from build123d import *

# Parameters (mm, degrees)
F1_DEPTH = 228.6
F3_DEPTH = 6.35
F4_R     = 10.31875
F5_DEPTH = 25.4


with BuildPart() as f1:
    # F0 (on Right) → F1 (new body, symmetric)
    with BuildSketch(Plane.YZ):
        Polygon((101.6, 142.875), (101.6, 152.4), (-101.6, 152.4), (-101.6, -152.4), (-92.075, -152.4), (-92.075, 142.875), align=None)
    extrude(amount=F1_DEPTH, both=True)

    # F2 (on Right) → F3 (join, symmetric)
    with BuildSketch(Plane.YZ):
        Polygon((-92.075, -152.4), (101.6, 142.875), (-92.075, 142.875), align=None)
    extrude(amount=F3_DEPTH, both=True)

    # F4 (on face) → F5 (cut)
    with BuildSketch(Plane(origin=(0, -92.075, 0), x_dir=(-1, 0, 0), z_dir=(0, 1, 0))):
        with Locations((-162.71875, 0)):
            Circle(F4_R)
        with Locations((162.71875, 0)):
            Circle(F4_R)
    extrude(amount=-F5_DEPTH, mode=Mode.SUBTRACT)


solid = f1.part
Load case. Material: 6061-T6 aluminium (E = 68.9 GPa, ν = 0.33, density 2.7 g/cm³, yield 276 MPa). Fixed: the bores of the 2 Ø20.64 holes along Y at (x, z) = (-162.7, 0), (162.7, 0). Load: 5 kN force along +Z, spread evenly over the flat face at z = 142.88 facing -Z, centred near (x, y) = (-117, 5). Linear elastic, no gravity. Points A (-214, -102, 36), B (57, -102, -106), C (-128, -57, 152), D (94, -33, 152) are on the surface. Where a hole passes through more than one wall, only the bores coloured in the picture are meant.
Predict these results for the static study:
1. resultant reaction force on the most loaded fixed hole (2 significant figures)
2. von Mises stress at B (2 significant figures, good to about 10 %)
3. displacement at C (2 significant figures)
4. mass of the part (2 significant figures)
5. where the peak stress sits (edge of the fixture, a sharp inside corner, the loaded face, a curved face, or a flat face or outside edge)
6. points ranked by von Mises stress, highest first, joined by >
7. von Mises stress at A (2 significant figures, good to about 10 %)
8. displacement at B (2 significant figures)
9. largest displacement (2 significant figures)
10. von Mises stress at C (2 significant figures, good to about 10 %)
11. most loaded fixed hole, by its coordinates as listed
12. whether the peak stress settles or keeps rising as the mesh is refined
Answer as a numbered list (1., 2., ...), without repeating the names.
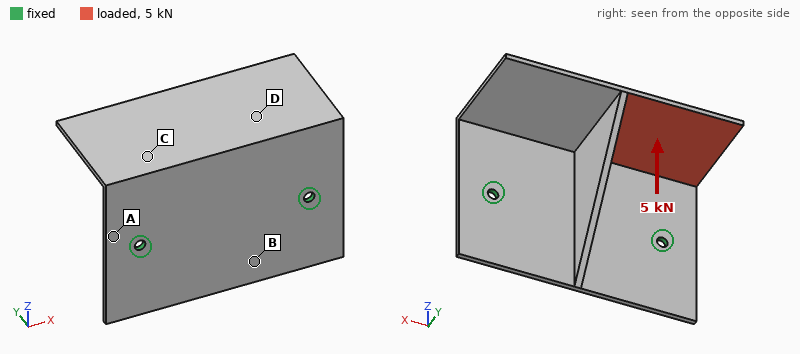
1. 4.3 kN
2. 21 MPa
3. 2.1 mm
4. 6.8 kg
5. edge of the fixture
6. A > C > B > D
7. 57 MPa
8. 1.3 mm
9. 5.9 mm
10. 35 MPa
11. (-162.7, 0)
12. keeps rising
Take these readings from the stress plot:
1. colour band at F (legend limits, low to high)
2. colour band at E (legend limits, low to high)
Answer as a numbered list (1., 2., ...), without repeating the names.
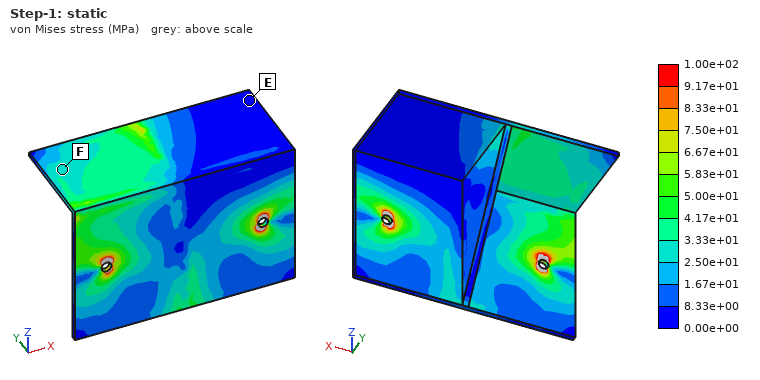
1. 2.50e+01 to 3.33e+01 MPa
2. 0.00e+00 to 8.33e+00 MPa
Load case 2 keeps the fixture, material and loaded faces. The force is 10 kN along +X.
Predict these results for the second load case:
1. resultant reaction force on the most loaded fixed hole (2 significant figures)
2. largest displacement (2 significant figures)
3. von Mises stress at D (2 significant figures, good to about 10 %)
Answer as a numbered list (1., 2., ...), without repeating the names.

1. 7.4 kN
2. 3.0 mm
3. 14 MPa
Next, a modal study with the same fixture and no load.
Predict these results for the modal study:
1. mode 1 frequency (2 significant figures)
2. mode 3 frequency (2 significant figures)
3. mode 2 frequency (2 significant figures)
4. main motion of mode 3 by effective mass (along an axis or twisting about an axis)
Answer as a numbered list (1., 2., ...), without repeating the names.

1. 100 Hz
2. 260 Hz
3. 180 Hz
4. along Y
